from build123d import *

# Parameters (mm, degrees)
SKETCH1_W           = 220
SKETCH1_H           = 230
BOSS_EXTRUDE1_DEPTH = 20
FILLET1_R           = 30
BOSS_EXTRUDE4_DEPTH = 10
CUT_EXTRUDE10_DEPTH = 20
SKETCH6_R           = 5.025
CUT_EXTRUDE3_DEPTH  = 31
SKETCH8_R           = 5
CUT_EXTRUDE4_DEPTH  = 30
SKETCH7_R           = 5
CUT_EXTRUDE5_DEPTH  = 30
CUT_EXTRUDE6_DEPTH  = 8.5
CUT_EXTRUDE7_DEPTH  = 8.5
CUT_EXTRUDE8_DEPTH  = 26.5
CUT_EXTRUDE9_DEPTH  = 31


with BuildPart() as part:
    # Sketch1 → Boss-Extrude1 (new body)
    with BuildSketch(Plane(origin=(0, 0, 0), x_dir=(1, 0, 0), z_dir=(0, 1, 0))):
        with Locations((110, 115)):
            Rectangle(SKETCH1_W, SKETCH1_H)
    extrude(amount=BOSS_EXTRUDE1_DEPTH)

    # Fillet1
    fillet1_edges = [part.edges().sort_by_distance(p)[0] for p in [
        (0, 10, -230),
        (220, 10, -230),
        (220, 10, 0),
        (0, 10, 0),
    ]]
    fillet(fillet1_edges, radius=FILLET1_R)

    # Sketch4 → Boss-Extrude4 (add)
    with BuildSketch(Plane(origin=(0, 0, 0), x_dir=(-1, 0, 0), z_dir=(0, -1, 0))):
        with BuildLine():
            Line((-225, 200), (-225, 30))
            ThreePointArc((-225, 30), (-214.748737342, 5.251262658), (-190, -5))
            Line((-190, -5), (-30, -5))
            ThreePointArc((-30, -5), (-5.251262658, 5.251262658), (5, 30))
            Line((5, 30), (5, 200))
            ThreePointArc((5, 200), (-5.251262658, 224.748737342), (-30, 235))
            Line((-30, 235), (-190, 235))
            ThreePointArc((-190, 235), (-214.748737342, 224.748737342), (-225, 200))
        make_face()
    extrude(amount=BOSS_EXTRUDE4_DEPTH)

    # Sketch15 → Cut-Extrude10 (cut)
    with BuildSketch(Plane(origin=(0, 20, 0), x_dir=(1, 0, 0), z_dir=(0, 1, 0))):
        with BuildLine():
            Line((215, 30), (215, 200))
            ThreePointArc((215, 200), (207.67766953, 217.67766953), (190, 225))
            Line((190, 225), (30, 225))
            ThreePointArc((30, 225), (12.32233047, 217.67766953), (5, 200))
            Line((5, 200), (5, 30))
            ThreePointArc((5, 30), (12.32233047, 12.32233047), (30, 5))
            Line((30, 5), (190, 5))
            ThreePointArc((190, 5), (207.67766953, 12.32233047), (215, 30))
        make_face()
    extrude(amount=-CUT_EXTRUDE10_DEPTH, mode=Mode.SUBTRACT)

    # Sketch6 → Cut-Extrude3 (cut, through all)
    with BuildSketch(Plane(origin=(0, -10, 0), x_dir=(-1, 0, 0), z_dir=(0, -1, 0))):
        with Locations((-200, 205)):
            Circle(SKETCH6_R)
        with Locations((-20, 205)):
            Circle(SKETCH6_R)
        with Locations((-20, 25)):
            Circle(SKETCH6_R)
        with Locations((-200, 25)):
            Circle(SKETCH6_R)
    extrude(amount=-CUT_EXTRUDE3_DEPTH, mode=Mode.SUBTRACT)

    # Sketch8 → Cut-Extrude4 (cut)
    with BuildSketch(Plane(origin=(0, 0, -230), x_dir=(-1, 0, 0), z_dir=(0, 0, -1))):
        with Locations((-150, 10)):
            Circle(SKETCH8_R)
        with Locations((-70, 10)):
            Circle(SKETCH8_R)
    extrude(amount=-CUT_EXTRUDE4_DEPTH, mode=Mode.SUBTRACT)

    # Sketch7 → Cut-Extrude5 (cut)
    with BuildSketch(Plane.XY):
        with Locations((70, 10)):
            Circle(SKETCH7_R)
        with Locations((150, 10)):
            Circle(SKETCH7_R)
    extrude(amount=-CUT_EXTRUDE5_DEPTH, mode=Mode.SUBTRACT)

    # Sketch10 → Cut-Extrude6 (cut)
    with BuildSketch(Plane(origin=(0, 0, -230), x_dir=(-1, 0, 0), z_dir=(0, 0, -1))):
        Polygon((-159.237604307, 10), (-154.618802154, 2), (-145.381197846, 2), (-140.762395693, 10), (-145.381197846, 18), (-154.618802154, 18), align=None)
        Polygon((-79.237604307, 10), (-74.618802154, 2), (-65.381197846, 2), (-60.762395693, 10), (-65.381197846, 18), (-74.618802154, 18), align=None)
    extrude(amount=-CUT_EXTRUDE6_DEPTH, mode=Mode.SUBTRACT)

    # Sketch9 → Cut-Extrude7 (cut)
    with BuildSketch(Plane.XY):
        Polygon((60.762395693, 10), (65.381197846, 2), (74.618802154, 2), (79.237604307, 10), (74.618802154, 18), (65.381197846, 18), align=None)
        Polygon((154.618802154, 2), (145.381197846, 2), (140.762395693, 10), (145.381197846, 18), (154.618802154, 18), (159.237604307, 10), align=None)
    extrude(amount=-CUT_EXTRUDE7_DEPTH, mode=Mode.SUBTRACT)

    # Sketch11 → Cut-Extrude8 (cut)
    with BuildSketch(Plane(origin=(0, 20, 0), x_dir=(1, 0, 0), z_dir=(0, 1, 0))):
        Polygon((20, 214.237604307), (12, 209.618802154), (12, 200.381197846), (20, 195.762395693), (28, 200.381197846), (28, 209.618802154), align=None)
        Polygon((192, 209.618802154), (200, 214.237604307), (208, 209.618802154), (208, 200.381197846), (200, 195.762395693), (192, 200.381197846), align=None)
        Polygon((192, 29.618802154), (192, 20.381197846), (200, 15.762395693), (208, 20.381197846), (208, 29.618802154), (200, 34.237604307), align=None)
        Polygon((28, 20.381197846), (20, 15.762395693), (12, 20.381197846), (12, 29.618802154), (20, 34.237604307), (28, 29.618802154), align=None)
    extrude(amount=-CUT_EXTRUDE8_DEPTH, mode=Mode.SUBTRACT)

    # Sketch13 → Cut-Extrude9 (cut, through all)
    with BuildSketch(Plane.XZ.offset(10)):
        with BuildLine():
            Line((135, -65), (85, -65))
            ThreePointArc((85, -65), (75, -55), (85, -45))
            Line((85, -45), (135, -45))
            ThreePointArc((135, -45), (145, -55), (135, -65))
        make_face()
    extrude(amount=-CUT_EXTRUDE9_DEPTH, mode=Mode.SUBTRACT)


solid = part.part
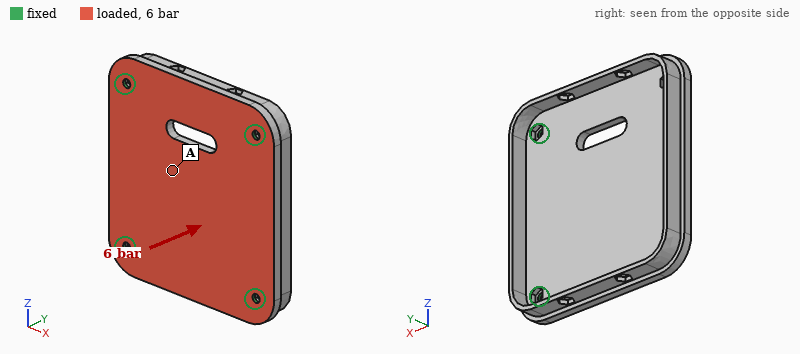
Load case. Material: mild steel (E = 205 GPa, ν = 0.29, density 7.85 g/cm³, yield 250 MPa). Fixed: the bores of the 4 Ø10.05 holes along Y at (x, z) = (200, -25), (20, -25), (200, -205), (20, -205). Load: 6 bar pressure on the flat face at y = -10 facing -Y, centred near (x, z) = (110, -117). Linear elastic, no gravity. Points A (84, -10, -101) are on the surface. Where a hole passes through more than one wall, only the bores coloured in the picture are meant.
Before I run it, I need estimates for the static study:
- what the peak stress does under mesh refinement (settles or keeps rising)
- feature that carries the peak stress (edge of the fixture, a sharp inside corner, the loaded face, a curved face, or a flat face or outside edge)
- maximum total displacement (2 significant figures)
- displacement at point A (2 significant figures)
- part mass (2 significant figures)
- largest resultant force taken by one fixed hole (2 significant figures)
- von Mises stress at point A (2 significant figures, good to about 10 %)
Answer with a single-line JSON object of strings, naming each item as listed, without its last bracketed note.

{"what the peak stress does under mesh refinement": "keeps rising", "feature that carries the peak stress": "edge of the fixture", "maximum total displacement": "0.28 mm", "displacement at point A": "0.26 mm", "part mass": "4.7 kg", "largest resultant force taken by one fixed hole": "13 kN", "von Mises stress at point A": "57 MPa"}
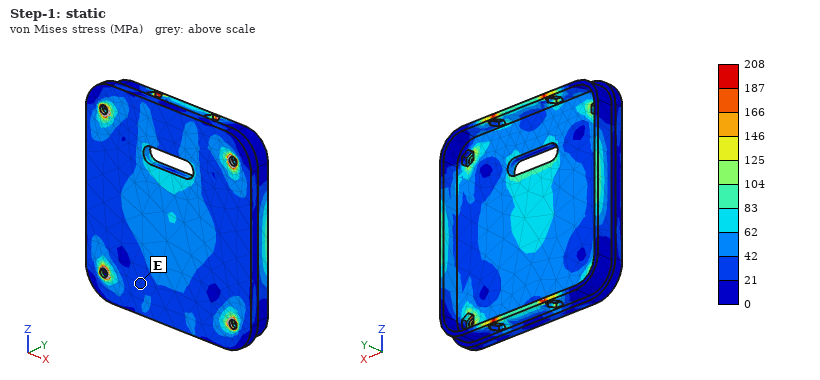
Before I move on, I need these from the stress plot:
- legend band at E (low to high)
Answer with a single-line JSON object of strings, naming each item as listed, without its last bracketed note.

{"legend band at E": "21 to 42 MPa"}
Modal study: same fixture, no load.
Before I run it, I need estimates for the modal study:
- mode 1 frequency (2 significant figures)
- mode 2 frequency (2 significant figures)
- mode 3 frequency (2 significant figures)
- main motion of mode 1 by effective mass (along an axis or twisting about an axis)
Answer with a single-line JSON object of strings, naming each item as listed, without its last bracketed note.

{"mode 1 frequency": "1000 Hz", "mode 2 frequency": "1700 Hz", "mode 3 frequency": "1700 Hz", "main motion of mode 1 by effective mass": "along Y"}
